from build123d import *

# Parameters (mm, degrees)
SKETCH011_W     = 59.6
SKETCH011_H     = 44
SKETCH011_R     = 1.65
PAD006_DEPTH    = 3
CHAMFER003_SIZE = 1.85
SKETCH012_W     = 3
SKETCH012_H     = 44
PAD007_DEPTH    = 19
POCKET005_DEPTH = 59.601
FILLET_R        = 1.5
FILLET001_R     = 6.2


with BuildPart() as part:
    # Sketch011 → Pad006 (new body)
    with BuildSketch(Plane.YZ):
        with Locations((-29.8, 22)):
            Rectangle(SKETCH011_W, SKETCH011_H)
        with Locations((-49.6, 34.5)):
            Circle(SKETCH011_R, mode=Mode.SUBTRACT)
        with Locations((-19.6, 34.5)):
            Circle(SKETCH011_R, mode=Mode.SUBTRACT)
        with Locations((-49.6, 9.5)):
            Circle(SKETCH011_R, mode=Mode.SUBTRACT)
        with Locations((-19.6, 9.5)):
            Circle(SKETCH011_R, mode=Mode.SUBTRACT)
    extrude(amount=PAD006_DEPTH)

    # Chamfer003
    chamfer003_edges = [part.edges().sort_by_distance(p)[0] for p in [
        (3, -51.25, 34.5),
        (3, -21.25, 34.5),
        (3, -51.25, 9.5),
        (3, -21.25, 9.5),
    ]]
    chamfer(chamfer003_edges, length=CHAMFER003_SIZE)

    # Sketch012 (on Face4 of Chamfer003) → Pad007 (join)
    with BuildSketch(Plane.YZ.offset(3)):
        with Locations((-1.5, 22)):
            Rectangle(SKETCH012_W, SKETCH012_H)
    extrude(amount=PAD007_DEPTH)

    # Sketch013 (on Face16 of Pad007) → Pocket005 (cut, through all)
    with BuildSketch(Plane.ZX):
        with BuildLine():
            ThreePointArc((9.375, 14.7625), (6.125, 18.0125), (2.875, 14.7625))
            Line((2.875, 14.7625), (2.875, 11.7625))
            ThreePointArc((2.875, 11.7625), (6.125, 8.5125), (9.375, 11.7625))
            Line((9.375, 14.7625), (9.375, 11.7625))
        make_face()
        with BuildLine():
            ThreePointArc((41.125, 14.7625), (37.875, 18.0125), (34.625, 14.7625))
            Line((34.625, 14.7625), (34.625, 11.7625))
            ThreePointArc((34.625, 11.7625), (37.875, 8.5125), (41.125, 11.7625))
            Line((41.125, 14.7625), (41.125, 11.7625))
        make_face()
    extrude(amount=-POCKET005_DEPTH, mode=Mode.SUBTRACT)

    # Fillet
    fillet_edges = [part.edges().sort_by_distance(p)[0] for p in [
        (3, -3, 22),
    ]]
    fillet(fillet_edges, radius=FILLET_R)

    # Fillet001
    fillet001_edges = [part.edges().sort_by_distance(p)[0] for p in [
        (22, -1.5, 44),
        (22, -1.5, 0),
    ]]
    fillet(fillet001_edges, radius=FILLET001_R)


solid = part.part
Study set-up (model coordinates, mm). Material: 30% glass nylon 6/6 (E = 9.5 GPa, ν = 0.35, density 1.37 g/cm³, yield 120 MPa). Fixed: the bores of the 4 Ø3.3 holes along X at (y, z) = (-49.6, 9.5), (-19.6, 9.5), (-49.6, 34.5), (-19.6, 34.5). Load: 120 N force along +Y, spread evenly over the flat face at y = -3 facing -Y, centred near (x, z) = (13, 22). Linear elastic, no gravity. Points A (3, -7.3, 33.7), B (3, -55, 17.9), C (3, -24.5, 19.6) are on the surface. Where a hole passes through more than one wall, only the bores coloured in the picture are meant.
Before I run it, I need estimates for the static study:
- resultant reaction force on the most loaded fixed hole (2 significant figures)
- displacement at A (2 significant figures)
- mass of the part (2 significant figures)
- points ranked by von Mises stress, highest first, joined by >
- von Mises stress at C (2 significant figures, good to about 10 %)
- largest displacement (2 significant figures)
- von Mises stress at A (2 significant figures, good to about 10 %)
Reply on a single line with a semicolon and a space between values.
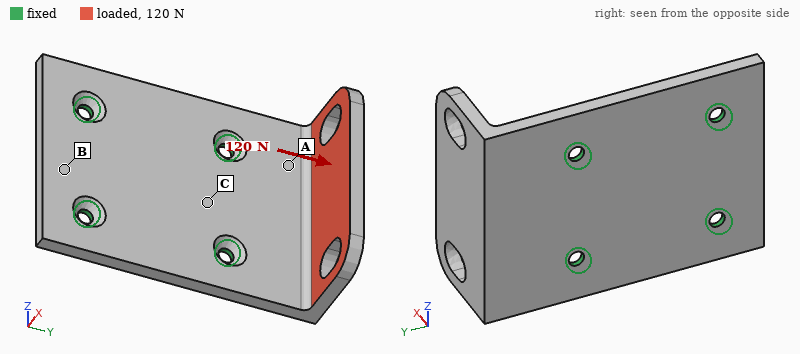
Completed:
86 N; 0.18 mm; 13 g; A > C > B; 9.9 MPa; 0.84 mm; 19 MPa
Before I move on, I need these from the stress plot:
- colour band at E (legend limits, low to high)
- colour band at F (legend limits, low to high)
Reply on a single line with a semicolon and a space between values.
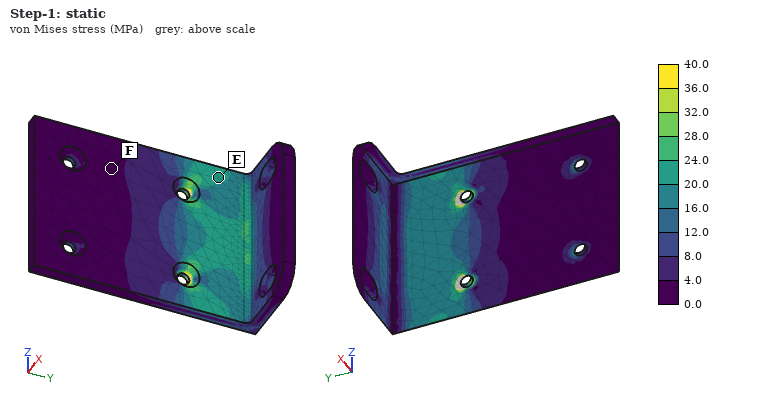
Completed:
20.0 to 24.0 MPa; 0.0 to 4.0 MPa
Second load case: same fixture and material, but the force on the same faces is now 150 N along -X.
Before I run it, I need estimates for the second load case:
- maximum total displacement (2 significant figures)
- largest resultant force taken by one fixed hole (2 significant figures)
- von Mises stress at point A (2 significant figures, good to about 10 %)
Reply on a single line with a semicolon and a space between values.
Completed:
0.77 mm; 160 N; 7.7 MPa
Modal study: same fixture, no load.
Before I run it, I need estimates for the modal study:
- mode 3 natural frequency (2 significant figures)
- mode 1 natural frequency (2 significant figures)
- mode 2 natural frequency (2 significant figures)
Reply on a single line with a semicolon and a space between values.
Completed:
3200 Hz; 1100 Hz; 1900 Hz
